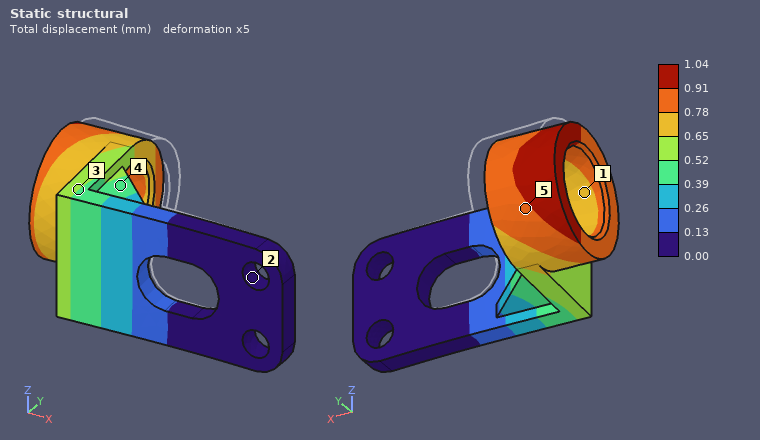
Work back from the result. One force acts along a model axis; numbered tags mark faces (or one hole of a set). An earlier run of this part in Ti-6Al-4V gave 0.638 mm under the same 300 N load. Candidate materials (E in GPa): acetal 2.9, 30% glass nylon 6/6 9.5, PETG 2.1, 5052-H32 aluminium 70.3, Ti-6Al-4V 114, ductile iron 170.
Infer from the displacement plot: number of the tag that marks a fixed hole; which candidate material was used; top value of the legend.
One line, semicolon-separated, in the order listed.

2; 5052-H32 aluminium; 1.04 mm
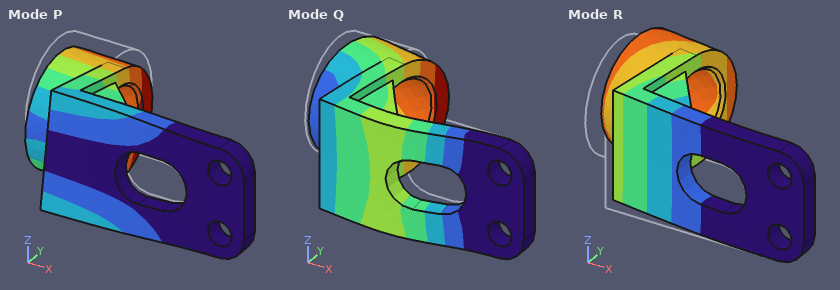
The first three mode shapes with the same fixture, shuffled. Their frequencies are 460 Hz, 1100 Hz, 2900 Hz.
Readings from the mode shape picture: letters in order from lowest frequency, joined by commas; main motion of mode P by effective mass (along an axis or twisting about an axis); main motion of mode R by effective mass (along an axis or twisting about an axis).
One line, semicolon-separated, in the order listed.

R, P, Q; along Z; along Y
